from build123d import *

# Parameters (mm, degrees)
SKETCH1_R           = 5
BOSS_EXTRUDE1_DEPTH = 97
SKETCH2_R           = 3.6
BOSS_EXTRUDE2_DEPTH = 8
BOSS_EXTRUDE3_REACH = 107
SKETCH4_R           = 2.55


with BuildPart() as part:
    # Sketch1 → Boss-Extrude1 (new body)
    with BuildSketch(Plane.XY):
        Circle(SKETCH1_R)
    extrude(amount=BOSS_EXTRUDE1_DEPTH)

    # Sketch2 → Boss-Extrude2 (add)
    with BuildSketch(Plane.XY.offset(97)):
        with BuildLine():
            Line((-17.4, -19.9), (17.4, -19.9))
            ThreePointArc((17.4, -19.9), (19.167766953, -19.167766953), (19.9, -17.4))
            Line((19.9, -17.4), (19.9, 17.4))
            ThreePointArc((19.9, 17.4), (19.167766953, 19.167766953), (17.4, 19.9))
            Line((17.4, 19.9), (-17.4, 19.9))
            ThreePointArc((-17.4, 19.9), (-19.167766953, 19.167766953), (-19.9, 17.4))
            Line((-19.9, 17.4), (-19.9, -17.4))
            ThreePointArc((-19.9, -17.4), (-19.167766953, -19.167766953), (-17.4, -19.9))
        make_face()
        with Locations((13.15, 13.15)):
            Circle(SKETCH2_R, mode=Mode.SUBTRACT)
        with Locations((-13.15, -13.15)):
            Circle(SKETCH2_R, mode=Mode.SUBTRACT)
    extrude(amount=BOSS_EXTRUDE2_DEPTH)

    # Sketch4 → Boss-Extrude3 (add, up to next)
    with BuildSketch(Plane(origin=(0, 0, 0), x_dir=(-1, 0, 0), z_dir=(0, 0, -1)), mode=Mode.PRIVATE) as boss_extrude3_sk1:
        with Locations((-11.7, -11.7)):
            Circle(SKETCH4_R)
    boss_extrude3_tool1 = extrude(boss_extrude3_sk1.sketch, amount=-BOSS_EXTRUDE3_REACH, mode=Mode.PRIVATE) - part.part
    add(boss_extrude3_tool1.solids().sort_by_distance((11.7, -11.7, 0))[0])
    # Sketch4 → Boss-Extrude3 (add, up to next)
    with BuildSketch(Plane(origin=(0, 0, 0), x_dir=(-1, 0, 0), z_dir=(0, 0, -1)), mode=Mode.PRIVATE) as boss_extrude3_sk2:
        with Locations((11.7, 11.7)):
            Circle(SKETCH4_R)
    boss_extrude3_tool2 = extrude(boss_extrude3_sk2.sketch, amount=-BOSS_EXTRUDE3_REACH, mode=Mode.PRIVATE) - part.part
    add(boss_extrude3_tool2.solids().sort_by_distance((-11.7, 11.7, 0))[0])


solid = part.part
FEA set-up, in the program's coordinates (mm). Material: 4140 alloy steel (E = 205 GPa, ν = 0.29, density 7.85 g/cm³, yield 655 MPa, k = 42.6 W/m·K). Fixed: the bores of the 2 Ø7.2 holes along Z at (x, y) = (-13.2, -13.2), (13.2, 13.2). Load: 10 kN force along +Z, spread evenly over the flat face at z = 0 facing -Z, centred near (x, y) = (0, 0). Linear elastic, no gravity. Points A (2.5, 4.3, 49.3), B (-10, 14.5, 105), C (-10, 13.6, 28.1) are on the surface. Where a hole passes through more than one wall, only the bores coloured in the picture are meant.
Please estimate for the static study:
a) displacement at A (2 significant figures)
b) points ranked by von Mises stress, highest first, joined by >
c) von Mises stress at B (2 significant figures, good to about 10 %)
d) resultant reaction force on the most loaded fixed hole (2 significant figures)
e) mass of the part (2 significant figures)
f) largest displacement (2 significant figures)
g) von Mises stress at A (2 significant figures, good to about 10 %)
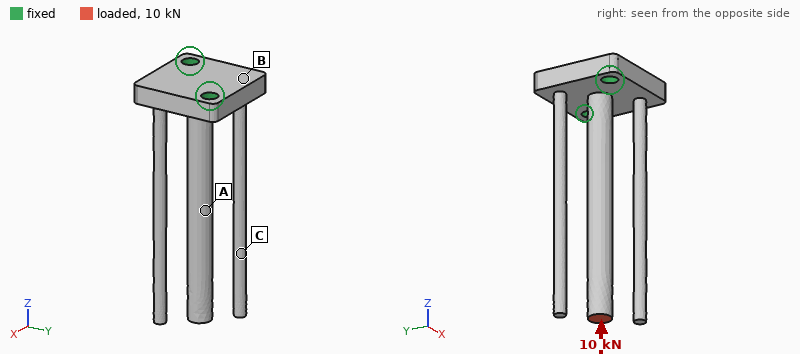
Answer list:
44 µm
A > B > C
42 MPa
5.0 kN
180 g
74 µm
130 MPa
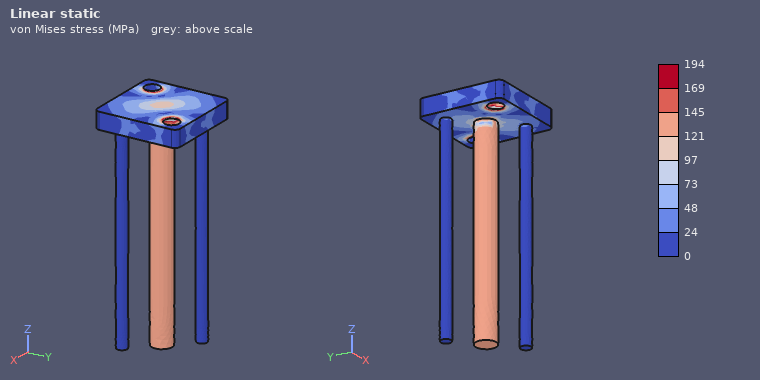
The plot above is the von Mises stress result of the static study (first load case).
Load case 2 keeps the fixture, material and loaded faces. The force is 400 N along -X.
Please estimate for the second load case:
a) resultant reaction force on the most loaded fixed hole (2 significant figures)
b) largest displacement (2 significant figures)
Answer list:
1.1 kN
1.4 mm
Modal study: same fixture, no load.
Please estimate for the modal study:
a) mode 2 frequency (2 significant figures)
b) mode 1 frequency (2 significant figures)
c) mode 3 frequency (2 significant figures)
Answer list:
370 Hz
370 Hz
380 Hz
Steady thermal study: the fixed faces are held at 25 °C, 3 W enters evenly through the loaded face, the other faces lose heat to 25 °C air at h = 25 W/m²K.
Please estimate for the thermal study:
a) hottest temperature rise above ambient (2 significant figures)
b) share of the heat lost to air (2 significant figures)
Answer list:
54 K
62 %
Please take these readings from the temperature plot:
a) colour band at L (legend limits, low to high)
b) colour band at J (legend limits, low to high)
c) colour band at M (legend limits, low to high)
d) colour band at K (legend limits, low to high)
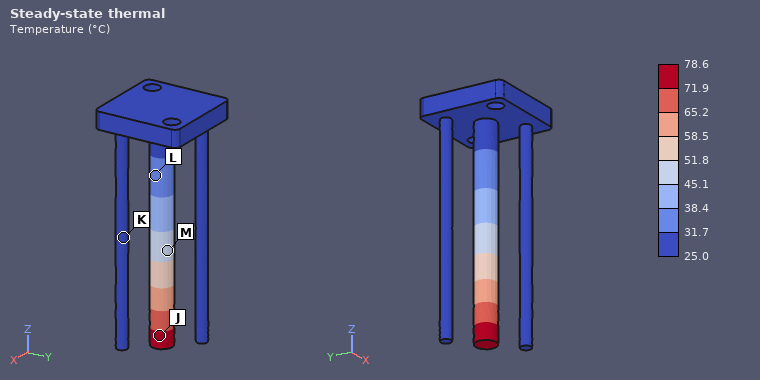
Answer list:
31.7 to 38.4 °C
71.9 to 78.6 °C
45.1 to 51.8 °C
25.0 to 31.7 °C
